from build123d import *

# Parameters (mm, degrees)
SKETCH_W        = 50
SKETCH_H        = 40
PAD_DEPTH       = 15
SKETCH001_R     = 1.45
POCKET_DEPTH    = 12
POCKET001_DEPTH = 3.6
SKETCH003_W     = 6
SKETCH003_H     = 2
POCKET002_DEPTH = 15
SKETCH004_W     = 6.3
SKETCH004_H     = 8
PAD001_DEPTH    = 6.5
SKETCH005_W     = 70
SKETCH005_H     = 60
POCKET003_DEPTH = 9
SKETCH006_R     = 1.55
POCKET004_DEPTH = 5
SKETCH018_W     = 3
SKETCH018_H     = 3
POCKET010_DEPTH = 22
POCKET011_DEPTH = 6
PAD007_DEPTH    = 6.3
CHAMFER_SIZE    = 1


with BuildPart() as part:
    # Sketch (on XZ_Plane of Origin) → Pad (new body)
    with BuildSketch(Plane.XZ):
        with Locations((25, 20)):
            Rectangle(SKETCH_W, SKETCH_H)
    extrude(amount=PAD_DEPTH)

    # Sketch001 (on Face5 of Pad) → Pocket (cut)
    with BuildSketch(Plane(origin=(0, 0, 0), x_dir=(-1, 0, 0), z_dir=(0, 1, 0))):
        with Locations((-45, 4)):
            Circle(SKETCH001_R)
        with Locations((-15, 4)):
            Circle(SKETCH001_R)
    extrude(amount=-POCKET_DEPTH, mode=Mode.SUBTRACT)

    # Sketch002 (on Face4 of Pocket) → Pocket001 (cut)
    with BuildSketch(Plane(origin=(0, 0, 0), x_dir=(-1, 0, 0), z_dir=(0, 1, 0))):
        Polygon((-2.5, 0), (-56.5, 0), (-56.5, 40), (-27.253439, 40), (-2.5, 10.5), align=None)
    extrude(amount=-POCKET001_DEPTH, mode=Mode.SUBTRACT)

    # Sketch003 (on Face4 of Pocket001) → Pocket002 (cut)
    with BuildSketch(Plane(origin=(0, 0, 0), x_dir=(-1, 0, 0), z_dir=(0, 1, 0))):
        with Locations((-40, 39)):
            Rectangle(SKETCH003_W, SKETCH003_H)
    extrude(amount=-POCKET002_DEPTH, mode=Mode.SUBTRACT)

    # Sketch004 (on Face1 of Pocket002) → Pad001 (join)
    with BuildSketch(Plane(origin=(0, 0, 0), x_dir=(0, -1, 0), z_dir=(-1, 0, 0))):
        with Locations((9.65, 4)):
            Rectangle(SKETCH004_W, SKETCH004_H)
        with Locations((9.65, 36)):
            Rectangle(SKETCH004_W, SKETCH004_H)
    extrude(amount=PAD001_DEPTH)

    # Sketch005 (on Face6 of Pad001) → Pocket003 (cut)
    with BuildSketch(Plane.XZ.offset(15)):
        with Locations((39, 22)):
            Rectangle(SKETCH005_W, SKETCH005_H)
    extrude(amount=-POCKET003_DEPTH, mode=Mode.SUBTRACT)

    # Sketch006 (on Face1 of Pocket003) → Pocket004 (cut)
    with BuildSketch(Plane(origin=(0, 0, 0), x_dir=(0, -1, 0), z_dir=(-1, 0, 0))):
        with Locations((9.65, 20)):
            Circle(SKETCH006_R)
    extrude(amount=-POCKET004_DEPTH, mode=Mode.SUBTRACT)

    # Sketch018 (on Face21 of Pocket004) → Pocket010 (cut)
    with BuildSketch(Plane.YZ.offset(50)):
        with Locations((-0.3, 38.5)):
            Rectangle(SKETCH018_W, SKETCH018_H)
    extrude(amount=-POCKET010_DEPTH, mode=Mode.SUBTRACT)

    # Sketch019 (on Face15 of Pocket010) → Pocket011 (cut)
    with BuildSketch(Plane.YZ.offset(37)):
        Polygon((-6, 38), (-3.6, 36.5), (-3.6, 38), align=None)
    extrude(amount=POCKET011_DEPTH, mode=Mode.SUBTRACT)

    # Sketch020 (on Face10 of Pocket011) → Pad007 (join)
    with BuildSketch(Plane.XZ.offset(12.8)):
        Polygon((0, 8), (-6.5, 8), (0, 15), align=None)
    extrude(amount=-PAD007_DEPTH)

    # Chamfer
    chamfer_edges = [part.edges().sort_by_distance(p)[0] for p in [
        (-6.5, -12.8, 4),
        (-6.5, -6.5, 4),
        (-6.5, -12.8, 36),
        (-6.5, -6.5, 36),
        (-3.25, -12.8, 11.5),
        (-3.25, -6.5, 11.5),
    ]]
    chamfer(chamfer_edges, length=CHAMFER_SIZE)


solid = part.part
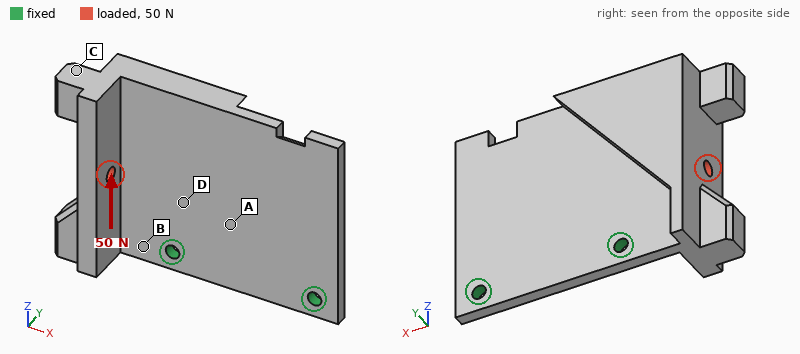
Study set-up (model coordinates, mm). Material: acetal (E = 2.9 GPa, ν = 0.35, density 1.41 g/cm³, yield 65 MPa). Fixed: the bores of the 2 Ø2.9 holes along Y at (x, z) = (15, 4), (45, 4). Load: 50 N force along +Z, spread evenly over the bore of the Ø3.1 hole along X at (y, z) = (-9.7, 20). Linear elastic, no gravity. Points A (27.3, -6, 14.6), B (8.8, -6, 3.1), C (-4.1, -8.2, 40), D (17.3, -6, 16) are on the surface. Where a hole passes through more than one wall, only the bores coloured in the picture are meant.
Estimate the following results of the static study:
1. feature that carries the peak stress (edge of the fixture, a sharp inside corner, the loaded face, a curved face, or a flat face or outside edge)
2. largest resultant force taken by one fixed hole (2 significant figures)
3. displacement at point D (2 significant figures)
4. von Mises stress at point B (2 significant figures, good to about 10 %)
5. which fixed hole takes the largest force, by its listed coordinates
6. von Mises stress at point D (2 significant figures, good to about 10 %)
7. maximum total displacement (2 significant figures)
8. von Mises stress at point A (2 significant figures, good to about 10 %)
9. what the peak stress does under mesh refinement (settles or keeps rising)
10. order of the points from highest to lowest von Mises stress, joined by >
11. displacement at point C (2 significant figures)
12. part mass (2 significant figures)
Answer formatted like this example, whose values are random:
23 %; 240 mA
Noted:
edge of the fixture; 70 N; 0.14 mm; 9.5 MPa; (15, 4); 3.2 MPa; 0.81 mm; 2.4 MPa; keeps rising; B > D > A > C; 0.78 mm; 12 g
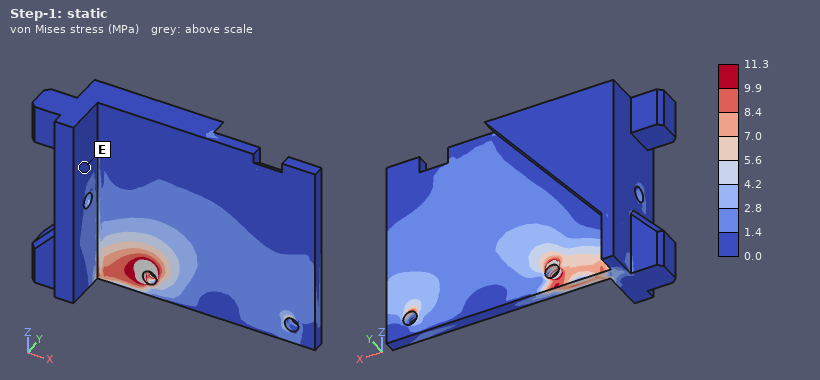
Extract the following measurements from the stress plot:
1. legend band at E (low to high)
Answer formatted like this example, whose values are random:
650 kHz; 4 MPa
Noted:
0.0 to 1.4 MPa
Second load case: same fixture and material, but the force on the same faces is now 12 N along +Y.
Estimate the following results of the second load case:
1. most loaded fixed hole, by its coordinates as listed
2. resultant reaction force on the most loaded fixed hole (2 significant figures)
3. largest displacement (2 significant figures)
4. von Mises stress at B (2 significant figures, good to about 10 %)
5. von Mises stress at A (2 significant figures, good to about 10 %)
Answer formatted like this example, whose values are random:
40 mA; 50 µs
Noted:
(15, 4); 15 N; 0.76 mm; 6.9 MPa; 2.3 MPa
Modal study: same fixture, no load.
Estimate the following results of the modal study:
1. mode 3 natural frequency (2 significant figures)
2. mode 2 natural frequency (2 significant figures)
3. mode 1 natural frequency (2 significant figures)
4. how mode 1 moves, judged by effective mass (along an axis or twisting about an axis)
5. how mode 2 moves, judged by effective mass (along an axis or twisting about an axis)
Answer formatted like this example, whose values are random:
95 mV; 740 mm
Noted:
1300 Hz; 580 Hz; 270 Hz; along Y; twisting about Z
